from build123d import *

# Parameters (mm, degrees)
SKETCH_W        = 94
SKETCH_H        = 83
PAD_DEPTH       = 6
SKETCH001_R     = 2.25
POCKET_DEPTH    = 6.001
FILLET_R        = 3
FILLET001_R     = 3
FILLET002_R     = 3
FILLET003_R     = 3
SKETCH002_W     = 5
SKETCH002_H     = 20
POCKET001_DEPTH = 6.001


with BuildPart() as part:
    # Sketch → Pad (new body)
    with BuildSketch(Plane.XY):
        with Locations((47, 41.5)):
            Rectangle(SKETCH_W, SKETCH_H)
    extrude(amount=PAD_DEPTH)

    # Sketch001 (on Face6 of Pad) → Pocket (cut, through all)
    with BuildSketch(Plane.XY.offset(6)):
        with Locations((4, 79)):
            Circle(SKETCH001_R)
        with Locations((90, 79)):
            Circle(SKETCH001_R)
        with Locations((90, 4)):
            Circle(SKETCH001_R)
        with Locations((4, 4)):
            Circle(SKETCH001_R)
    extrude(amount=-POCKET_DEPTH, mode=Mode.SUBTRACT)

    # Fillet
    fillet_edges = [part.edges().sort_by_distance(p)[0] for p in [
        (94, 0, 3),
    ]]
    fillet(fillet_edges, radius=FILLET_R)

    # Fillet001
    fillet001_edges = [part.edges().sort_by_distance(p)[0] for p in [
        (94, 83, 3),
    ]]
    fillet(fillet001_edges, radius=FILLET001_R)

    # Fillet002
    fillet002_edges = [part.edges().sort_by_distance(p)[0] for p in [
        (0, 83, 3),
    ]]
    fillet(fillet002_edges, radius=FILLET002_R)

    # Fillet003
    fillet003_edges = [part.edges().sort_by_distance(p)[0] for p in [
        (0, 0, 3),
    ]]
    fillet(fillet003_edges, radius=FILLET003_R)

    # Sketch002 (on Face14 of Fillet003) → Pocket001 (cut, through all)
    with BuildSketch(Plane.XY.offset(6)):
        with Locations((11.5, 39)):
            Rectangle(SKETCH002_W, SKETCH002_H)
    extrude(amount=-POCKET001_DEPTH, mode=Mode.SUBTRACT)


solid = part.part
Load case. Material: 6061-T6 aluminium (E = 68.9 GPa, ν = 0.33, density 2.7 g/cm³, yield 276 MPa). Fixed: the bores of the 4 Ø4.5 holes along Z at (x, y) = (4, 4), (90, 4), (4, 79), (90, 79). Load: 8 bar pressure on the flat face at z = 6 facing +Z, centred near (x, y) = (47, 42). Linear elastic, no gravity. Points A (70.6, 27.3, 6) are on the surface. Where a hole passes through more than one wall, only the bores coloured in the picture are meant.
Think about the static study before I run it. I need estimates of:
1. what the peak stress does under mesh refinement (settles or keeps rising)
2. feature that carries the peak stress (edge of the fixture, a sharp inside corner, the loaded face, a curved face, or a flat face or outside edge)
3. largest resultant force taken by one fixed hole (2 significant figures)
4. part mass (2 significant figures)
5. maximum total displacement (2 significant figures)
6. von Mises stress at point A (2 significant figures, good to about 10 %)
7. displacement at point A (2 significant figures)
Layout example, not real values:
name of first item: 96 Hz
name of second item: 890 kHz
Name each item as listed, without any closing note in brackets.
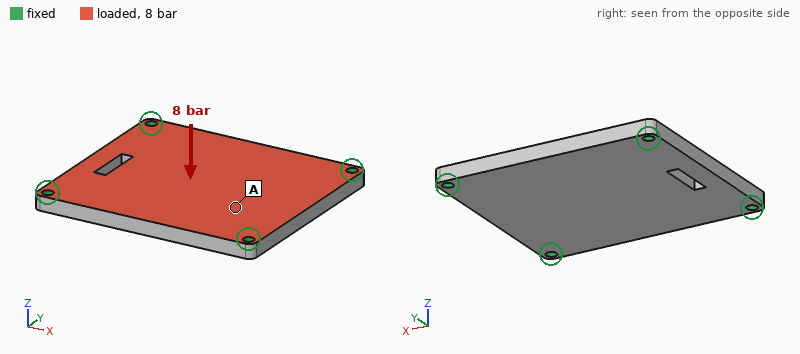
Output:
what the peak stress does under mesh refinement: keeps rising
feature that carries the peak stress: edge of the fixture
largest resultant force taken by one fixed hole: 1.5 kN
part mass: 120 g
maximum total displacement: 0.23 mm
von Mises stress at point A: 35 MPa
displacement at point A: 0.16 mm
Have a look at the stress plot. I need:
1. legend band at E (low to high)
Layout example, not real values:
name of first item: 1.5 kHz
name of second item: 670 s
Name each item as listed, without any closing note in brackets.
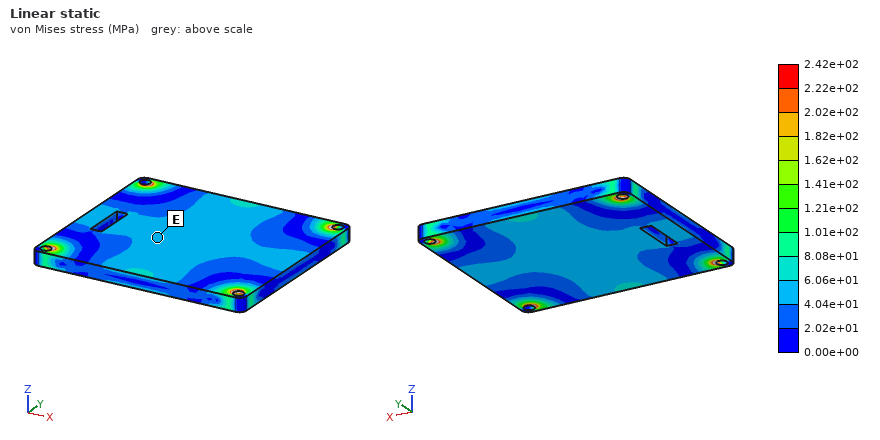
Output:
legend band at E: 4.04e+01 to 6.06e+01 MPa
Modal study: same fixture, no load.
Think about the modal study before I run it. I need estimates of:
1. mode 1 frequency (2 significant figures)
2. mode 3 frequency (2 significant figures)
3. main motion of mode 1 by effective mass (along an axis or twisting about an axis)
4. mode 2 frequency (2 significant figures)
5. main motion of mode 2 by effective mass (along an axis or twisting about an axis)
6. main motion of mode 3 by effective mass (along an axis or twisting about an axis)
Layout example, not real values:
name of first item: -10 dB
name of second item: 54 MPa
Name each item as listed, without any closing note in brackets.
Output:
mode 1 frequency: 2800 Hz
mode 3 frequency: 5500 Hz
main motion of mode 1 by effective mass: along Z
mode 2 frequency: 4700 Hz
main motion of mode 2 by effective mass: twisting about X
main motion of mode 3 by effective mass: twisting about Y
